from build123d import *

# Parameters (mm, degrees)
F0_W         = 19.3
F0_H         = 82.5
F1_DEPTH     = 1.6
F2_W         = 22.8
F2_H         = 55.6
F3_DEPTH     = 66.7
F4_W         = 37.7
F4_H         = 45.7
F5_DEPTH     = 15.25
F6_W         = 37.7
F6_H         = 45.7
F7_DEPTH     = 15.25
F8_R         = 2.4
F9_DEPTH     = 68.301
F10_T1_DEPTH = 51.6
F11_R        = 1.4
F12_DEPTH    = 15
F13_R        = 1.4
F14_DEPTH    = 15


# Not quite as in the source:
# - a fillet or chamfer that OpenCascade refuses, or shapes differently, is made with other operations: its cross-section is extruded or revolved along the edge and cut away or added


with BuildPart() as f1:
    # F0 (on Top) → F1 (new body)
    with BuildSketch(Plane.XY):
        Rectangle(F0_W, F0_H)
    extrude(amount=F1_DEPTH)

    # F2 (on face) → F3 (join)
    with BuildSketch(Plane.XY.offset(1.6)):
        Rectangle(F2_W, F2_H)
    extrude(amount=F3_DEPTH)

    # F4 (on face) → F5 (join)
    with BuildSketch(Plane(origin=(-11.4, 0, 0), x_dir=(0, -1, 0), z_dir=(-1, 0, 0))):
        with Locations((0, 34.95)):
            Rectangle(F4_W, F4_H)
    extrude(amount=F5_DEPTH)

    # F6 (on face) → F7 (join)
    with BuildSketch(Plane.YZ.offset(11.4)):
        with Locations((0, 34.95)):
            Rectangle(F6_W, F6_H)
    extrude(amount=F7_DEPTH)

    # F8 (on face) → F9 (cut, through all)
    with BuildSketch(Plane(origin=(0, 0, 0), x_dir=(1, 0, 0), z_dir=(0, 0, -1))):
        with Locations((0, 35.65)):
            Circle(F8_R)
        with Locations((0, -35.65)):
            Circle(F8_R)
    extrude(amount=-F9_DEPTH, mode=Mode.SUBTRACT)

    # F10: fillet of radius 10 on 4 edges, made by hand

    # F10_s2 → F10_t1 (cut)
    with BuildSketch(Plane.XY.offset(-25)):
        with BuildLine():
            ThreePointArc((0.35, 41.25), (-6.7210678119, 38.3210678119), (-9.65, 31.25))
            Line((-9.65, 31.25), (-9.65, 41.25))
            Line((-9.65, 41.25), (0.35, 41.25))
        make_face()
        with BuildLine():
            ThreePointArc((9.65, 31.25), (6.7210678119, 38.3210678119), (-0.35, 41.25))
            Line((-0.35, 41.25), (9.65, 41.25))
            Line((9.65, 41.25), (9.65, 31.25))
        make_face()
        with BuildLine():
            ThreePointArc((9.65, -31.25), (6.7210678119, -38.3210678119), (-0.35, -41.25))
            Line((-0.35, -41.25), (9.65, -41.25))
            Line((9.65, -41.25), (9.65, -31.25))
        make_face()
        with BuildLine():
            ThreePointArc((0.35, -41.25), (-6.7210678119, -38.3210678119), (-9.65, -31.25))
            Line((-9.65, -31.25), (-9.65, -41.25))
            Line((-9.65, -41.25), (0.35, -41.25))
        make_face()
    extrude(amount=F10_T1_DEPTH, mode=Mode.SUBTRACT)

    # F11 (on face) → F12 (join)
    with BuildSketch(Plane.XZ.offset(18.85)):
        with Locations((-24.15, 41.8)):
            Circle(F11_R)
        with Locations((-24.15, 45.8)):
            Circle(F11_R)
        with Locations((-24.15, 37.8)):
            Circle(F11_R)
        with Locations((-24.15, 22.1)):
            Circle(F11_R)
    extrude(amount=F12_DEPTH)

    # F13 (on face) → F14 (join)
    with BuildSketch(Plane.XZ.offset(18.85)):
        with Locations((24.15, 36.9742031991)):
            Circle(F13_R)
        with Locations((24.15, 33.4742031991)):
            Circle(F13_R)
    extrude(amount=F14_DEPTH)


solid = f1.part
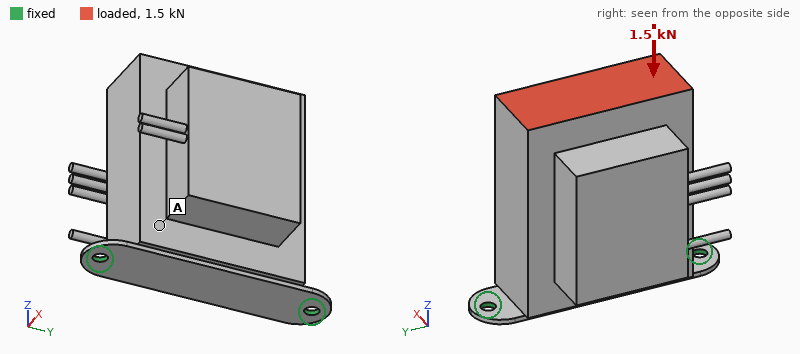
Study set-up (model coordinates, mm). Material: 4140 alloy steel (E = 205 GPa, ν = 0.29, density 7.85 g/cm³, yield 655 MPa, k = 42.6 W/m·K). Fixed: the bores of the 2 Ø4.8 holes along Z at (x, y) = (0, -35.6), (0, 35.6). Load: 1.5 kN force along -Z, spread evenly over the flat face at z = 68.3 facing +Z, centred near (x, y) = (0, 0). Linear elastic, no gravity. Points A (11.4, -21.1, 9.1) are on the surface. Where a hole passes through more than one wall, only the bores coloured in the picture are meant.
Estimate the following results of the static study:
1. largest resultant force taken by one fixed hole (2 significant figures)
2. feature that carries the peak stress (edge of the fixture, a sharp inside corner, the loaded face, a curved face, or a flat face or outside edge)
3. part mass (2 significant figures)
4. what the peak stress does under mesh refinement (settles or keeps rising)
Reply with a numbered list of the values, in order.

1. 860 N
2. edge of the fixture
3. 1.1 kg
4. keeps rising
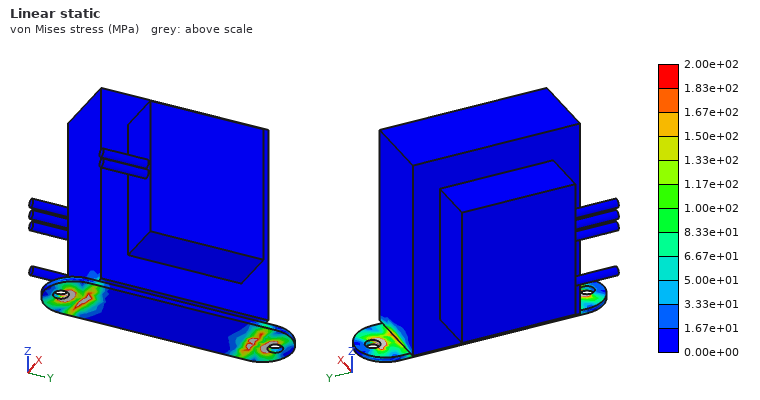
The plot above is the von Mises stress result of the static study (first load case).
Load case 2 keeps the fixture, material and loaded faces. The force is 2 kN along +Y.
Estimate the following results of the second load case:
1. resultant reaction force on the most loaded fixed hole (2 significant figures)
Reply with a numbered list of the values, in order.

1. 2.4 kN
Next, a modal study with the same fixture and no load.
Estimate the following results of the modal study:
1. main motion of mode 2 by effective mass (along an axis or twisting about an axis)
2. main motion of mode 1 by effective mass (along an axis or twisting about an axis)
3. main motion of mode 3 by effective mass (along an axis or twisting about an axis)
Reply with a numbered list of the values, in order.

1. along Y
2. along X
3. along Z
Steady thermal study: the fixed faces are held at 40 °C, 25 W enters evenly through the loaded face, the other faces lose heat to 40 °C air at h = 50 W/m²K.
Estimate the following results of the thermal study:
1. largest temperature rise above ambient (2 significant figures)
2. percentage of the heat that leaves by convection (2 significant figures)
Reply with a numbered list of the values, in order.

1. 33 K
2. 82 %
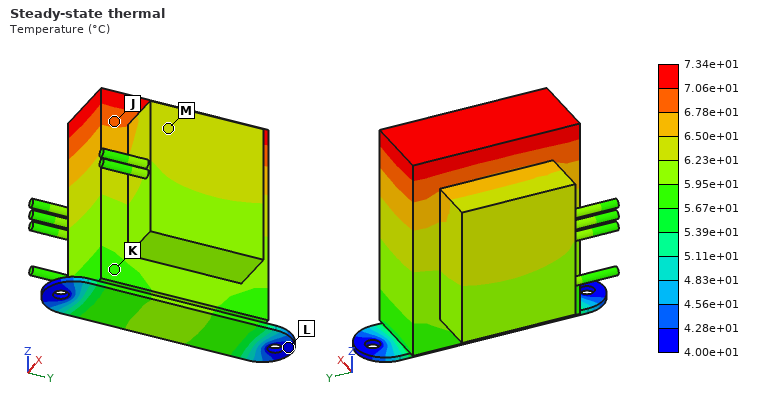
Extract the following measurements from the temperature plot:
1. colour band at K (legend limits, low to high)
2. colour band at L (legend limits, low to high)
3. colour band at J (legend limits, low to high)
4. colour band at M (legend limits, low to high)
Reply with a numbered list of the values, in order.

1. 5.67e+01 to 5.95e+01 °C
2. 4.00e+01 to 4.28e+01 °C
3. 6.78e+01 to 7.06e+01 °C
4. 6.23e+01 to 6.50e+01 °C
